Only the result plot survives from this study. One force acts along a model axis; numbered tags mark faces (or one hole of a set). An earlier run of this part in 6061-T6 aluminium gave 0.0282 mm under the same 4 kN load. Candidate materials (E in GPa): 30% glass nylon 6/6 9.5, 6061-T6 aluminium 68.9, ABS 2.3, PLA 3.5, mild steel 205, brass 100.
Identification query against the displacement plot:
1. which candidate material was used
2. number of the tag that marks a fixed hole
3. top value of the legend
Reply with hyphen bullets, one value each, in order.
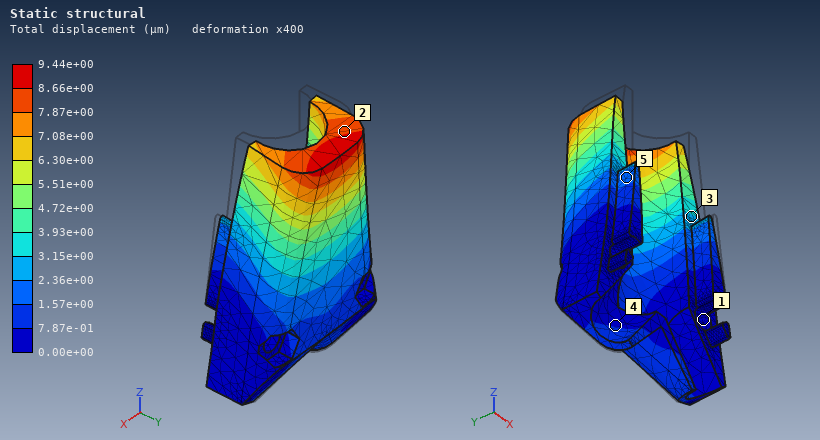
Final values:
- mild steel
- 1
- 9.44e+00 µm
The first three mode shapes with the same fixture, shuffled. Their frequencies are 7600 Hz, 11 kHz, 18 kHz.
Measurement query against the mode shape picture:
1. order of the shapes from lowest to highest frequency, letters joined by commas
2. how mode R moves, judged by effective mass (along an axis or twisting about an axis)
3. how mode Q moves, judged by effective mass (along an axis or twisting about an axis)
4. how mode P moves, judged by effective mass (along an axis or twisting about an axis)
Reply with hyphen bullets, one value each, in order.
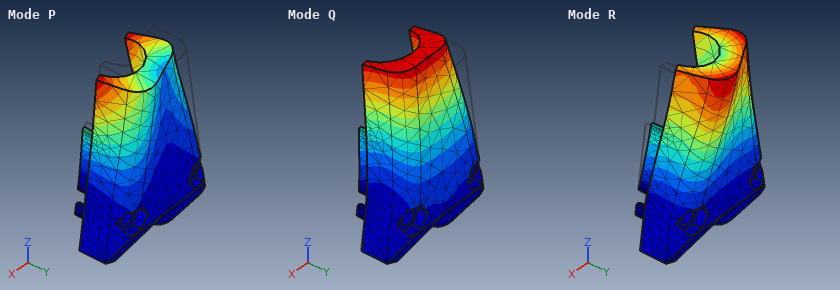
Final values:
- Q, P, R
- along X
- along Y
- along X
